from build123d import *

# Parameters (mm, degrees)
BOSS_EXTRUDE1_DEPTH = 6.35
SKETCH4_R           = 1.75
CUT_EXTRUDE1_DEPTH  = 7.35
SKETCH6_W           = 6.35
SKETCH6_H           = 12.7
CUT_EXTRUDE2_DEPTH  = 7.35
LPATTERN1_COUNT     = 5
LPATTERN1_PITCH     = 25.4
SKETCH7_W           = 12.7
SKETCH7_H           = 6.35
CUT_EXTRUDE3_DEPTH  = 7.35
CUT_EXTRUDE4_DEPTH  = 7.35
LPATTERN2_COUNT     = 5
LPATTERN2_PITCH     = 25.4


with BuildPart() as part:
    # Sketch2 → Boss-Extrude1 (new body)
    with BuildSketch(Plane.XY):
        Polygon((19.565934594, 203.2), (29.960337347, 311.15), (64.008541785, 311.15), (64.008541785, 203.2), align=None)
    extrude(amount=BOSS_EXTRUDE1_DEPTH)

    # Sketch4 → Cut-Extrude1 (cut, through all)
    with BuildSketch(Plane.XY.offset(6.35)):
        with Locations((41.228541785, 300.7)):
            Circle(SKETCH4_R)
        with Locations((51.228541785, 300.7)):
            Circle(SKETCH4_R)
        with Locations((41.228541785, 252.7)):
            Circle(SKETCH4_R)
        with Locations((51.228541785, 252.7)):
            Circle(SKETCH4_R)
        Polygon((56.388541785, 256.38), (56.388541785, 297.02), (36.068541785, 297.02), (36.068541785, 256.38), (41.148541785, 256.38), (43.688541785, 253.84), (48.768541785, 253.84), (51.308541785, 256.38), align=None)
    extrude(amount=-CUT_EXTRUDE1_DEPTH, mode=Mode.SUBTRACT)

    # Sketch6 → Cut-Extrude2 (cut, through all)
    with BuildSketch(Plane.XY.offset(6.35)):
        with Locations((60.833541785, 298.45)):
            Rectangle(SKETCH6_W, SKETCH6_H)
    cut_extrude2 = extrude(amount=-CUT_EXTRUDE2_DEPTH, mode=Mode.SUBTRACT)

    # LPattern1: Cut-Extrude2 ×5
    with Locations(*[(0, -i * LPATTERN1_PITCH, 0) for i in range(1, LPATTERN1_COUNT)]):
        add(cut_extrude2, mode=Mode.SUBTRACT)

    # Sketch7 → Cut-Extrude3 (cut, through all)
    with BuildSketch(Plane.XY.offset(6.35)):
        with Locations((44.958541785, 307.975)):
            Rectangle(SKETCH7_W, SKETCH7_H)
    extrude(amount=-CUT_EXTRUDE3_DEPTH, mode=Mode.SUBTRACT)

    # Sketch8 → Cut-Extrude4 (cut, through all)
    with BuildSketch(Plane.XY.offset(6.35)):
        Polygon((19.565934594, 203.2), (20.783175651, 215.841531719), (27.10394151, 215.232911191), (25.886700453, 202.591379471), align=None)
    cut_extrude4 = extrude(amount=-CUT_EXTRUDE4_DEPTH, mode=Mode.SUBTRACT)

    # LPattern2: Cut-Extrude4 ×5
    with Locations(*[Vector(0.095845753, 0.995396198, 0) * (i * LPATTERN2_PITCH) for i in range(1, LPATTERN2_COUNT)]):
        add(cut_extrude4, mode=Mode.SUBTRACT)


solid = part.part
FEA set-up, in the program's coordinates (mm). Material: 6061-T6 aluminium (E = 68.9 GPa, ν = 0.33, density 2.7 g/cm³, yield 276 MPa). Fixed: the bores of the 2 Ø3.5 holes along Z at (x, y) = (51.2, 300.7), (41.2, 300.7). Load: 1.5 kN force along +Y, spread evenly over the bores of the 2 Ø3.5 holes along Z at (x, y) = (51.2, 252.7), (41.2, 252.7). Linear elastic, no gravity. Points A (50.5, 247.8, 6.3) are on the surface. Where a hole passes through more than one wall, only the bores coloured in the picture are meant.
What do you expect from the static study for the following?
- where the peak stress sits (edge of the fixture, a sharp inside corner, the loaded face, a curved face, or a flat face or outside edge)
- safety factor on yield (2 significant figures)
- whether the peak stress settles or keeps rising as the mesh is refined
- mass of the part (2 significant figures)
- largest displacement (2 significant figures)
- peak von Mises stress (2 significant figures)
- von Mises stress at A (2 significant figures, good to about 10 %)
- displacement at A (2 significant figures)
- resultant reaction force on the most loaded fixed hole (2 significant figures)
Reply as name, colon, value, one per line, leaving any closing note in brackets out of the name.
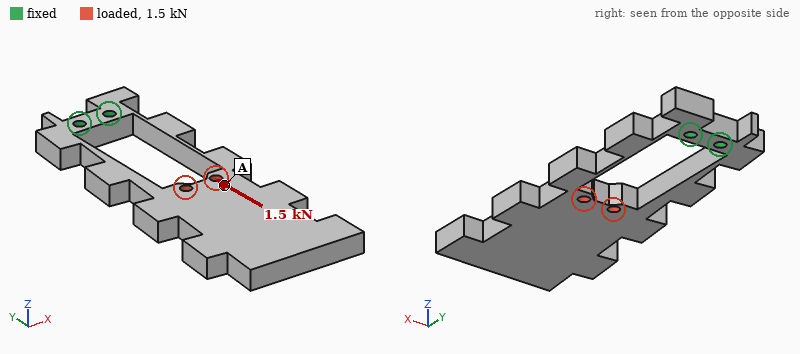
where the peak stress sits: a flat face or outside edge
safety factor on yield: 2.2
whether the peak stress settles or keeps rising as the mesh is refined: settles
mass of the part: 44 g
largest displacement: 83 µm
peak von Mises stress: 130 MPa
von Mises stress at A: 14 MPa
displacement at A: 78 µm
resultant reaction force on the most loaded fixed hole: 770 N
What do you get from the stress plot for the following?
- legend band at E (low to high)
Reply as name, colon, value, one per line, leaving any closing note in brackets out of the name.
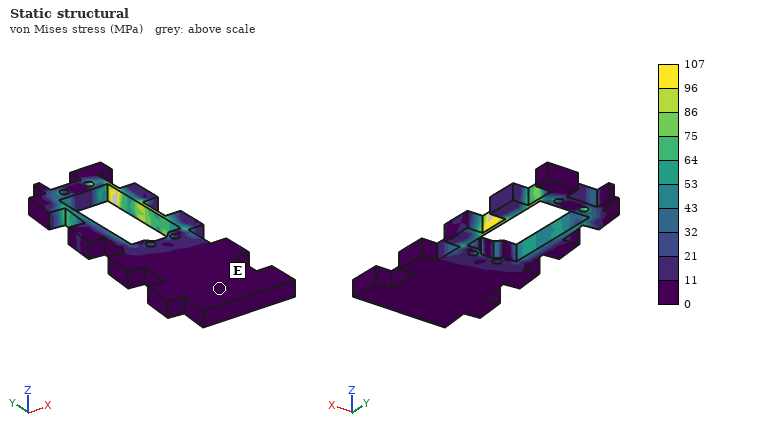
legend band at E: 0 to 11 MPa
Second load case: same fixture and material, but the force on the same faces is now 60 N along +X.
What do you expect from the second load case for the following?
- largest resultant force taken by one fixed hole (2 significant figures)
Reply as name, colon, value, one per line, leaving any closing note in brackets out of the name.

largest resultant force taken by one fixed hole: 150 N
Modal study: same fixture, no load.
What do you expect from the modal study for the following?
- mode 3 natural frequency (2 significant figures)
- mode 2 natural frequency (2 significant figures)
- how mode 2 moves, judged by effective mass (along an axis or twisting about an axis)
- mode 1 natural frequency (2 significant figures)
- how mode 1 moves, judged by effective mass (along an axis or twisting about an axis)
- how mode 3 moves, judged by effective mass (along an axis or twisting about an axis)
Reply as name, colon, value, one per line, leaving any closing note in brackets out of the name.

mode 3 natural frequency: 830 Hz
mode 2 natural frequency: 400 Hz
how mode 2 moves, judged by effective mass: along X
mode 1 natural frequency: 210 Hz
how mode 1 moves, judged by effective mass: along Z
how mode 3 moves, judged by effective mass: twisting about Y
